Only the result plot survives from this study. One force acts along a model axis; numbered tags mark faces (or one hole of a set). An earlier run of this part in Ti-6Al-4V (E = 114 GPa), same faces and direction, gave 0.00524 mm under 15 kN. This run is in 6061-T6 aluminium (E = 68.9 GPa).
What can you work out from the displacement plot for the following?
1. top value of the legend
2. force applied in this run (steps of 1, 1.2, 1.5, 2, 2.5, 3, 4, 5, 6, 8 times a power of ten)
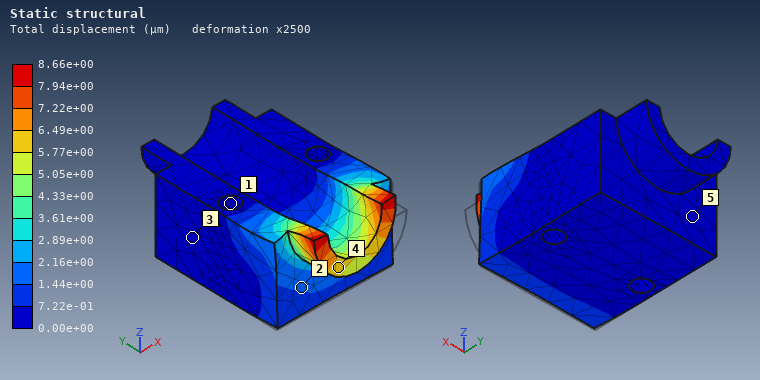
8.66e+00 µm
15 kN
